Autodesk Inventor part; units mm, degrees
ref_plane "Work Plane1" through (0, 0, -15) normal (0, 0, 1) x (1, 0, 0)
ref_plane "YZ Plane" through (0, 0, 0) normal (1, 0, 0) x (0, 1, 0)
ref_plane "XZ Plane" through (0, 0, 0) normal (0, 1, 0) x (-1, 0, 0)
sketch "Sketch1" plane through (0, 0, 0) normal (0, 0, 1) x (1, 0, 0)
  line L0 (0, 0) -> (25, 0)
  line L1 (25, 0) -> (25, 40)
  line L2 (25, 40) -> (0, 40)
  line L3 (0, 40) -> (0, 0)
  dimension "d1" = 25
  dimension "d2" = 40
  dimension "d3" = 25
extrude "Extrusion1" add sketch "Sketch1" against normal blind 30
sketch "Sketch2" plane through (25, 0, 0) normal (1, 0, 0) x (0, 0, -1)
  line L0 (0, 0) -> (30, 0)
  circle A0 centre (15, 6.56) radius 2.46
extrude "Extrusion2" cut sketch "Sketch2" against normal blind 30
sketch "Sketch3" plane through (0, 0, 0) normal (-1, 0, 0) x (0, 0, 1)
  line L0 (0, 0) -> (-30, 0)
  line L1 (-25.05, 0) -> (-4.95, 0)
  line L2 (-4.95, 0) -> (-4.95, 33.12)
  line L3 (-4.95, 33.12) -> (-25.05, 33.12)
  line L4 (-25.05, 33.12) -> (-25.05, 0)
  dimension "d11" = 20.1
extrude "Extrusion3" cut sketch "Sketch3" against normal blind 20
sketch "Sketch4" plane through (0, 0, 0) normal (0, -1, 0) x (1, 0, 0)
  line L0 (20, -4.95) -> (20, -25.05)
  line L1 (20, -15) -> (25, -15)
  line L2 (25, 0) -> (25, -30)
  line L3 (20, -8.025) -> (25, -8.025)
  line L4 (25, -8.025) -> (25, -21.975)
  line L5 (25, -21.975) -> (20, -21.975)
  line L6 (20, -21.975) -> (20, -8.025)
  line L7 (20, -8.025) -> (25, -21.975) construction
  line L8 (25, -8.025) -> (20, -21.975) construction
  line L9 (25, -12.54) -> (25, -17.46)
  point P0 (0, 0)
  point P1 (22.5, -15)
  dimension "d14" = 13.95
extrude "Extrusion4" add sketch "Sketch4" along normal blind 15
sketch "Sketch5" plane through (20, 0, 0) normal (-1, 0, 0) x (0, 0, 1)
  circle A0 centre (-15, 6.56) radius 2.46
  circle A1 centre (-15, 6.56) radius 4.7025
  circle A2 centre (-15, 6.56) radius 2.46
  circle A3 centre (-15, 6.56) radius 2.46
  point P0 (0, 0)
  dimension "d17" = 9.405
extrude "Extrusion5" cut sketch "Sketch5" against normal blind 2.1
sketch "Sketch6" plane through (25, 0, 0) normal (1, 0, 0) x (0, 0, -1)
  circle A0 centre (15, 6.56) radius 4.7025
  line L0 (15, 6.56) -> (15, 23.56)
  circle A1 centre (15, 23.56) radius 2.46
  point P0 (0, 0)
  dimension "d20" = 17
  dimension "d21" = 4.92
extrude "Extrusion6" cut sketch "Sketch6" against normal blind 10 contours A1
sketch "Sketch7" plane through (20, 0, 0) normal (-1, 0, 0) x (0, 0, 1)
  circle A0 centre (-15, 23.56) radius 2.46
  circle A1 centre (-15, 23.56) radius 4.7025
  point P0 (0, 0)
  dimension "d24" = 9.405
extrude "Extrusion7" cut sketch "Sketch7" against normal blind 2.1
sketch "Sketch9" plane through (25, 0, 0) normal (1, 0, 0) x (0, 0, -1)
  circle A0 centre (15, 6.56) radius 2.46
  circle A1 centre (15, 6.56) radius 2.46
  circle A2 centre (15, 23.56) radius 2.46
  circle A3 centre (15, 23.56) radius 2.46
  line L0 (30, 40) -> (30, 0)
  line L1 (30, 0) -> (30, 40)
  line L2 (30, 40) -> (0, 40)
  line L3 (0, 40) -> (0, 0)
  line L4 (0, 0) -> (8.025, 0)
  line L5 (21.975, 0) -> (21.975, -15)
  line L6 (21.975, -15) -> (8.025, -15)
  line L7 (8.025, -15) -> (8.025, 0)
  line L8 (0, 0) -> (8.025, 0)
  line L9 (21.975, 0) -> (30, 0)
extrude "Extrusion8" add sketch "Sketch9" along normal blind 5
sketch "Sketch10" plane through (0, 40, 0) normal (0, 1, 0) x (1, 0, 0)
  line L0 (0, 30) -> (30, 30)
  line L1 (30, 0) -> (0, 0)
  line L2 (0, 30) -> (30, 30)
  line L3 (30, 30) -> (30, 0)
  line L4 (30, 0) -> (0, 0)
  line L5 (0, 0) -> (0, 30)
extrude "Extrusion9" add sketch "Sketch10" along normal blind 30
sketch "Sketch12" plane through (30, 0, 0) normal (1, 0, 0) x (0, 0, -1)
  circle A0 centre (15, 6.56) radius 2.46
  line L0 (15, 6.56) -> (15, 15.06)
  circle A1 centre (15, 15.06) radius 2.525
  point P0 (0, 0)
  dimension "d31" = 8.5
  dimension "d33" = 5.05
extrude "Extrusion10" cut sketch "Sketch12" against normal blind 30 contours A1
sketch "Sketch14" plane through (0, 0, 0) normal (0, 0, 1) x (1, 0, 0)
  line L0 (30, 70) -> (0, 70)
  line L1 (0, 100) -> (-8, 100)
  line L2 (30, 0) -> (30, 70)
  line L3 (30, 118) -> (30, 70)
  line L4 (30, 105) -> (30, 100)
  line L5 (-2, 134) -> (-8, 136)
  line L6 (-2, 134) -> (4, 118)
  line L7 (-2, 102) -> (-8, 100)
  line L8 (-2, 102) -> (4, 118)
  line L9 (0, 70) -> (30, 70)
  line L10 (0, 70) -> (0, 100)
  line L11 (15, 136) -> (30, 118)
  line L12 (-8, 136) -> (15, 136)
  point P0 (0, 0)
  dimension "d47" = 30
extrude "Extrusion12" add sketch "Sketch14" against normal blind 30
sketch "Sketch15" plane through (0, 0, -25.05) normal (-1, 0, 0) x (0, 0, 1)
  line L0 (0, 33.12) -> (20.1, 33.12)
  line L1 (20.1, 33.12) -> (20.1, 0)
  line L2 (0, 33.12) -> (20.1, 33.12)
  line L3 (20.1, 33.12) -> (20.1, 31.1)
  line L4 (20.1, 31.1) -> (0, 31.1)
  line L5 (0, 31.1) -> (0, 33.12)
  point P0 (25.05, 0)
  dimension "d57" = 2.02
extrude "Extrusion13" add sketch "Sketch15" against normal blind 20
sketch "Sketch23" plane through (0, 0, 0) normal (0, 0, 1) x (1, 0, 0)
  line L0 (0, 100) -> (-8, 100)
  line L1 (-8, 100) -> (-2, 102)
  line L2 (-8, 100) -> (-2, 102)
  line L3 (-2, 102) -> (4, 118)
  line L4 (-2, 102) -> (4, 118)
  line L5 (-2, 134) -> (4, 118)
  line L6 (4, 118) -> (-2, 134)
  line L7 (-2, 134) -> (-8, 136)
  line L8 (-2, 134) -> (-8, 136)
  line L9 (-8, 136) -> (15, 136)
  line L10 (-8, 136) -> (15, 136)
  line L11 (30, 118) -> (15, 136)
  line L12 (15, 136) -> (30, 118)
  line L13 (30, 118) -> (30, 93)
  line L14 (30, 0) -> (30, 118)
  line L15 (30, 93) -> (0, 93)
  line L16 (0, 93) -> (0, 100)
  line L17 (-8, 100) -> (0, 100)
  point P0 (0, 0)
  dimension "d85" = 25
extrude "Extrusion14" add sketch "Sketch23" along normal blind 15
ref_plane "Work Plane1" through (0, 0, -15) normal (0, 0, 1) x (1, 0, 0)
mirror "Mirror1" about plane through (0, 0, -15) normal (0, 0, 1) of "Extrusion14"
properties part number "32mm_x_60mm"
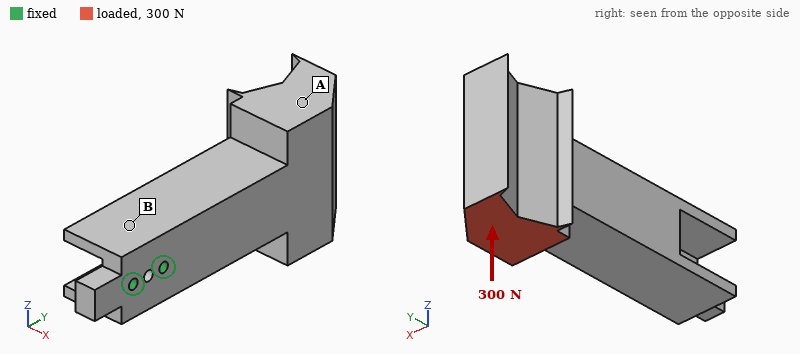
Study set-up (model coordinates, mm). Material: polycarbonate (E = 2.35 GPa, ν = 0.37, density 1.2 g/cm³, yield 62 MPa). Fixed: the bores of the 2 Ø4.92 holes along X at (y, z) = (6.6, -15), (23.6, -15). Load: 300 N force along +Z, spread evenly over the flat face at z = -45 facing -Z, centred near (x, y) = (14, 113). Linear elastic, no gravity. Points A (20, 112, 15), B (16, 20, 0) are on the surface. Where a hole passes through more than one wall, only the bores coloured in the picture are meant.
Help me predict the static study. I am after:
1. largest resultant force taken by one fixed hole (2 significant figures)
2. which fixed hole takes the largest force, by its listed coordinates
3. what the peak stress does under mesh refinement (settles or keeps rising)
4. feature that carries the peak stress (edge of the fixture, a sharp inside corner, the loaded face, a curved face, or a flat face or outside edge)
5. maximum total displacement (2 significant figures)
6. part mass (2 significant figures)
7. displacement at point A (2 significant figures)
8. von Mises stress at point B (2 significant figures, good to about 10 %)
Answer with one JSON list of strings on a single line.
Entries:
["1.5 kN", "(23.6, -15)", "keeps rising", "edge of the fixture", "2.0 mm", "170 g", "1.5 mm", "7.6 MPa"]
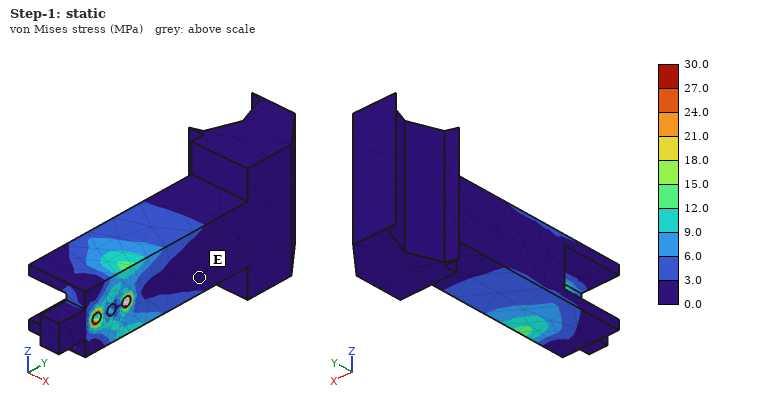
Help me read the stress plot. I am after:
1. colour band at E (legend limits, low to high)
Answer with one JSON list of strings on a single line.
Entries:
["0.0 to 3.0 MPa"]
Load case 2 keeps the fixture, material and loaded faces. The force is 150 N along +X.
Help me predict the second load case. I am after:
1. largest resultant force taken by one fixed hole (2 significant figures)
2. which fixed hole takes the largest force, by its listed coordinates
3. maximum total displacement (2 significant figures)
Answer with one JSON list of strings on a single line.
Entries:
["680 N", "(23.6, -15)", "1.6 mm"]
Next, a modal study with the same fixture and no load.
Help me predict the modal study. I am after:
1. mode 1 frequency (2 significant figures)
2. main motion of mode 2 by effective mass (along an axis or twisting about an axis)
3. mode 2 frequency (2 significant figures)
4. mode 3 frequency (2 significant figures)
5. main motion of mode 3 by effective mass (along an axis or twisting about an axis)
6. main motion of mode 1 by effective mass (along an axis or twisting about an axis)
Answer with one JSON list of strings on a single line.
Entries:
["200 Hz", "along Z", "230 Hz", "550 Hz", "twisting about Y", "along X"]
